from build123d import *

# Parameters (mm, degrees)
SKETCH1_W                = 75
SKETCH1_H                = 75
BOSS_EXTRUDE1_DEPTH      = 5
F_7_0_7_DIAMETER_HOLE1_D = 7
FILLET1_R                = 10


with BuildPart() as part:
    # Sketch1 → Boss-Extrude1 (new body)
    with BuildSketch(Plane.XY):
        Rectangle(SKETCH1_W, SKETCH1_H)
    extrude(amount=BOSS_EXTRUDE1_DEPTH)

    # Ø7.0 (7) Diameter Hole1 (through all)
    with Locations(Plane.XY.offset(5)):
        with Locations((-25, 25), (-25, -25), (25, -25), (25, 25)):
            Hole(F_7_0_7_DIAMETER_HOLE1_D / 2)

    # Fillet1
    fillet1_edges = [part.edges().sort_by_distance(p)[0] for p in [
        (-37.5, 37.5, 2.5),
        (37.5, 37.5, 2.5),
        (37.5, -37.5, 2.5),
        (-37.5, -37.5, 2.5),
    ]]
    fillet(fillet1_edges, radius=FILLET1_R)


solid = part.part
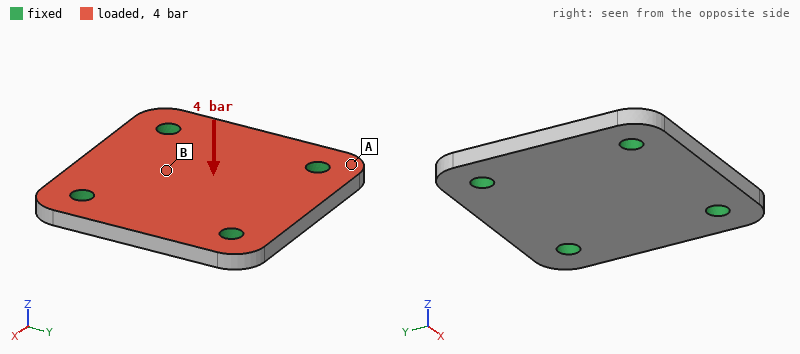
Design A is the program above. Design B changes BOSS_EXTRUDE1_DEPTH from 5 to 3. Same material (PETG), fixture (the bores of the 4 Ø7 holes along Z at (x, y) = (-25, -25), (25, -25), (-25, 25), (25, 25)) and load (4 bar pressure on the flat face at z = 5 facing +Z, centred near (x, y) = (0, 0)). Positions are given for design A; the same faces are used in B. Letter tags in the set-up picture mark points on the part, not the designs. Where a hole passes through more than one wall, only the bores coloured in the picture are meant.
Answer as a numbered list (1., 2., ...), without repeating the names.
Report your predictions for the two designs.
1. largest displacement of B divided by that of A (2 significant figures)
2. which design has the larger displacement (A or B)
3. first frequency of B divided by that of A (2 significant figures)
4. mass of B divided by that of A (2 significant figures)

1. 4.1
2. B
3. 0.64
4. 0.60
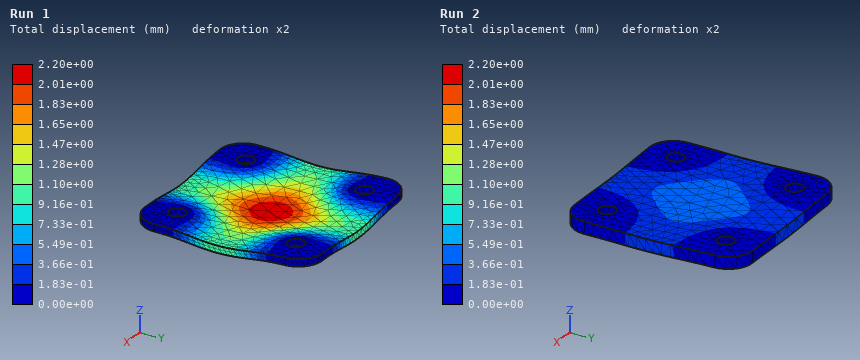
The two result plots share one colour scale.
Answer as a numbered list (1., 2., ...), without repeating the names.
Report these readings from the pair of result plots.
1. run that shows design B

1. Run 1
